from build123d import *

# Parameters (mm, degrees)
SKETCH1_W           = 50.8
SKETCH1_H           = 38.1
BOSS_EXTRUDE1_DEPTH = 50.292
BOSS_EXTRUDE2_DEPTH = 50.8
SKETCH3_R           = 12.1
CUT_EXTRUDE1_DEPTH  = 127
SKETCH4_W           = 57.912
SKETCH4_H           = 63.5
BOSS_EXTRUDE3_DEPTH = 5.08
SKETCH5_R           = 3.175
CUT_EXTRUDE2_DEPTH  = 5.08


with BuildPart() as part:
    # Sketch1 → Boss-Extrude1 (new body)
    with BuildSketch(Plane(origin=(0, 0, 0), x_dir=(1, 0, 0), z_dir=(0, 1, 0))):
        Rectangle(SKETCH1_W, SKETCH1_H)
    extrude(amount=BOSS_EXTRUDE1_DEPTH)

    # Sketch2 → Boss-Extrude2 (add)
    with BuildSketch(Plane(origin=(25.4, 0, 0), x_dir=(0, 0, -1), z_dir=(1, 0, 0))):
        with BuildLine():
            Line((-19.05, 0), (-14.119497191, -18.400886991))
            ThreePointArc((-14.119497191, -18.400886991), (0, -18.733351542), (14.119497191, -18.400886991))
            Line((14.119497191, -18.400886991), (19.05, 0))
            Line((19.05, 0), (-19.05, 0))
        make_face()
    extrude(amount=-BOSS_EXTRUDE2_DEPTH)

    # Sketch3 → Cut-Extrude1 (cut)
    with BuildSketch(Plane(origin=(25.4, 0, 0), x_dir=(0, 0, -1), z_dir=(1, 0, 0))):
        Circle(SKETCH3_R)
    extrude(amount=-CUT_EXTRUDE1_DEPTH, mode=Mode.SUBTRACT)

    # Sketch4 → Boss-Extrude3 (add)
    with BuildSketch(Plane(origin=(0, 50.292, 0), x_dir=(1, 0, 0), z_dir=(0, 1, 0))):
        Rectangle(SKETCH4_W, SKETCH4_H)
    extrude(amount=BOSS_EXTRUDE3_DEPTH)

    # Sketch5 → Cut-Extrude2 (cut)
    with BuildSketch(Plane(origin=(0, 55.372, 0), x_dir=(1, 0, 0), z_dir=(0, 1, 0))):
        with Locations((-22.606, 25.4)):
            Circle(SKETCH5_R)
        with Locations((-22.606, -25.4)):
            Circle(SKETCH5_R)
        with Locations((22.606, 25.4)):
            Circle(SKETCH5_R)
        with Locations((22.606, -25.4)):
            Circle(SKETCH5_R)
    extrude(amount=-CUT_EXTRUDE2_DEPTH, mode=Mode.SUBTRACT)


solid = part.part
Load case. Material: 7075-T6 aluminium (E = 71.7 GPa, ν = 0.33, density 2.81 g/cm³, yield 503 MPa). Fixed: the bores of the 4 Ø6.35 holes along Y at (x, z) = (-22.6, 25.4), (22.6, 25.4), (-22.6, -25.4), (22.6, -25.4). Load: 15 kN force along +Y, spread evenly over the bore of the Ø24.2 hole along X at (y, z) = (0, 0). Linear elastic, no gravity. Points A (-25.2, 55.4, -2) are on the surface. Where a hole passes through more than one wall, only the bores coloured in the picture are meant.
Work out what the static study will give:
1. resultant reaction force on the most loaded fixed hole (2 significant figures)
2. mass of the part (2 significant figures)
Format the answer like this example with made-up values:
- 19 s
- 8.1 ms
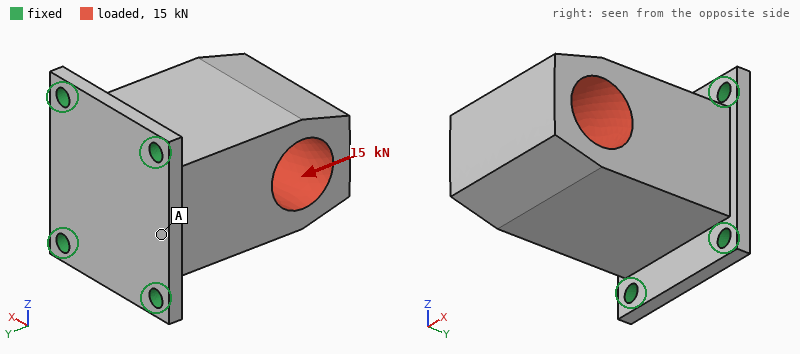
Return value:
- 4.1 kN
- 350 g
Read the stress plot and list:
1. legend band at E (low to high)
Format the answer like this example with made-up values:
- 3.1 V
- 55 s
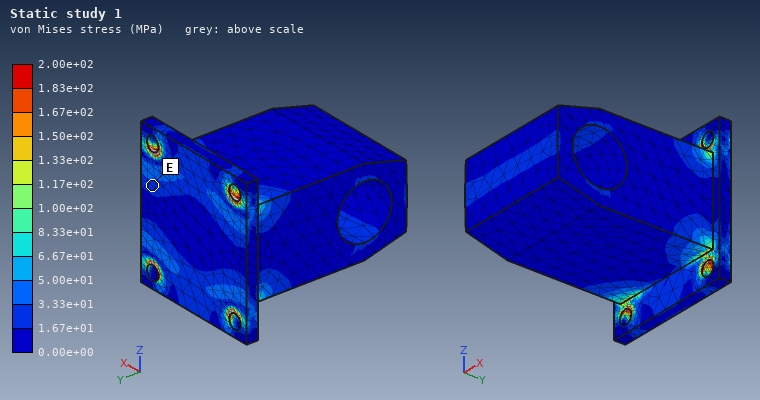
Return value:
- 1.67e+01 to 3.33e+01 MPa
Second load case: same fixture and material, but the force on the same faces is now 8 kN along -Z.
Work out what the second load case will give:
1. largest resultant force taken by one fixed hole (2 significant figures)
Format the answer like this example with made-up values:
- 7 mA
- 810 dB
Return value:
- 5.4 kN
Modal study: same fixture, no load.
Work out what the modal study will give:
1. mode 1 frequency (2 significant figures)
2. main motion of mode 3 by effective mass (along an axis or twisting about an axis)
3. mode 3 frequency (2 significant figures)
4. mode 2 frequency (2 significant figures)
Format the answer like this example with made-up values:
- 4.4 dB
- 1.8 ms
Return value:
- 3200 Hz
- along Y
- 6100 Hz
- 3200 Hz
